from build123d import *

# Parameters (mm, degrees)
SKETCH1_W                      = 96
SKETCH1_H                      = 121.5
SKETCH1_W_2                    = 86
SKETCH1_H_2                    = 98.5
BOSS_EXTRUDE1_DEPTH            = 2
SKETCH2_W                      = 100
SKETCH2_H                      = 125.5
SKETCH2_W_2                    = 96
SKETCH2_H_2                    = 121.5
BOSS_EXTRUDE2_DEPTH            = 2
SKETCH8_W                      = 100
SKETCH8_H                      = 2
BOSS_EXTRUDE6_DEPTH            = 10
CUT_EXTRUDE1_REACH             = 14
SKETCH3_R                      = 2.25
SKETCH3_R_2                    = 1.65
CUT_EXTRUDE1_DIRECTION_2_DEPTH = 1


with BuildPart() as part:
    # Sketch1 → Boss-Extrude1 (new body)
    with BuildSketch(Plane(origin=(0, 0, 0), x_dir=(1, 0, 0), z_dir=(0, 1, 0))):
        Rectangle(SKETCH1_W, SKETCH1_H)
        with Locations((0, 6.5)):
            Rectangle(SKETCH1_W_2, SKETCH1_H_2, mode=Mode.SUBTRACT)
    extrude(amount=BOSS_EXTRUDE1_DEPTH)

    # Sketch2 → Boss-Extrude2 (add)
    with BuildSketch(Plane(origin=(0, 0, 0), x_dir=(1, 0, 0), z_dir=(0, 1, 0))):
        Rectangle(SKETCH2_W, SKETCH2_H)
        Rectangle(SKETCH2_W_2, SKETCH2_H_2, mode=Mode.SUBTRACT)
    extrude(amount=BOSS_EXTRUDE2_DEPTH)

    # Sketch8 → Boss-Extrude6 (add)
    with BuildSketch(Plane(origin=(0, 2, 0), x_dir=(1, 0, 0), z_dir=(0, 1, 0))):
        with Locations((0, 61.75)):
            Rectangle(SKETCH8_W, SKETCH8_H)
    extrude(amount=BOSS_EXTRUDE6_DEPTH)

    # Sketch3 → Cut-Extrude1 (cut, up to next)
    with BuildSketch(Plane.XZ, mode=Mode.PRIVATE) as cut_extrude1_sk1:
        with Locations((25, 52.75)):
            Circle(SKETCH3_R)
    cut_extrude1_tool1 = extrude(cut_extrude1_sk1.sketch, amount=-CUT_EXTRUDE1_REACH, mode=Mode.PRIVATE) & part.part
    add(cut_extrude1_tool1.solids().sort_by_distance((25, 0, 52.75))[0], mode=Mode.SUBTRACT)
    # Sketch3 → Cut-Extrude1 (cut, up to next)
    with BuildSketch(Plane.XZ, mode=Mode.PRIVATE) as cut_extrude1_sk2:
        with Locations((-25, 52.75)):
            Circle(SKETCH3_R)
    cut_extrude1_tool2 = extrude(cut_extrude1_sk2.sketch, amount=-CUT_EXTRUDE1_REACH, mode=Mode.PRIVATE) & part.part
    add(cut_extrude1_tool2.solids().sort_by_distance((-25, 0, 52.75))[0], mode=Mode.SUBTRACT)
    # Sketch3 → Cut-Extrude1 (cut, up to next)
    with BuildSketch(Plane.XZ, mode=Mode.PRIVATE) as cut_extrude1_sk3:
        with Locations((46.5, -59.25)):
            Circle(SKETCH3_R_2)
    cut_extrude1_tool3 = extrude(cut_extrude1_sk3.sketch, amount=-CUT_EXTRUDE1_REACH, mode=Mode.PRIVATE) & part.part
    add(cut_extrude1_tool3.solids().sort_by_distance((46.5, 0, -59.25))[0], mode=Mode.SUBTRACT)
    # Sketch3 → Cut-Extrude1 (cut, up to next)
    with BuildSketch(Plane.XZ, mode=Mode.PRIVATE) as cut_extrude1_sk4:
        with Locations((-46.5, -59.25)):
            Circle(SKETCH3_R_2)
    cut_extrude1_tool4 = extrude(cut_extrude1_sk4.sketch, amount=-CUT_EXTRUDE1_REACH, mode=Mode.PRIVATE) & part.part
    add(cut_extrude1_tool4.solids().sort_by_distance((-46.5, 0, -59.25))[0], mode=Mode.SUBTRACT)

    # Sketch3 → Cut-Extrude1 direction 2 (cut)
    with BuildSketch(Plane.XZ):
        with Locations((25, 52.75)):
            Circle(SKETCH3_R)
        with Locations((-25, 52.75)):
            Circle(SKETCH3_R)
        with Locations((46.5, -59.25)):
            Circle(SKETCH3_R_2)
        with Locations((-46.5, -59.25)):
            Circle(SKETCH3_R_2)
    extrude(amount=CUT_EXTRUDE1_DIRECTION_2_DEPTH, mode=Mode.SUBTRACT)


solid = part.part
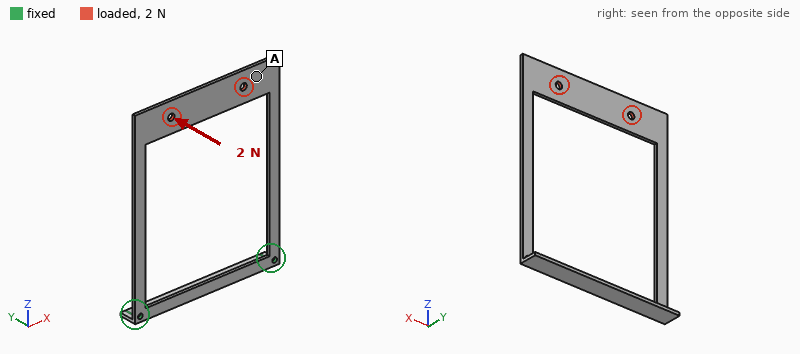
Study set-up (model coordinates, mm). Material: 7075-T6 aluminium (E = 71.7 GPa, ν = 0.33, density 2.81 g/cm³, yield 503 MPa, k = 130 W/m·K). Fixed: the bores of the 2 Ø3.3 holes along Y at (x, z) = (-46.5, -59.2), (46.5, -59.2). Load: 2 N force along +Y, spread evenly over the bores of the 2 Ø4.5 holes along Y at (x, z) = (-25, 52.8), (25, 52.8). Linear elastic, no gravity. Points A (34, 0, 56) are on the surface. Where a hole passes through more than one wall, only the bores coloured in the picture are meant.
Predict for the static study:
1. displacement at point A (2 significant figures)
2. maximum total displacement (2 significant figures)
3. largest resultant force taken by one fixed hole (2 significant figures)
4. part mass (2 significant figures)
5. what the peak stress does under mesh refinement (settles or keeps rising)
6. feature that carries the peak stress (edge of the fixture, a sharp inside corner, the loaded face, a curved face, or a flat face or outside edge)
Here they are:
1.4 mm
1.5 mm
1.0 N
28 g
keeps rising
edge of the fixture
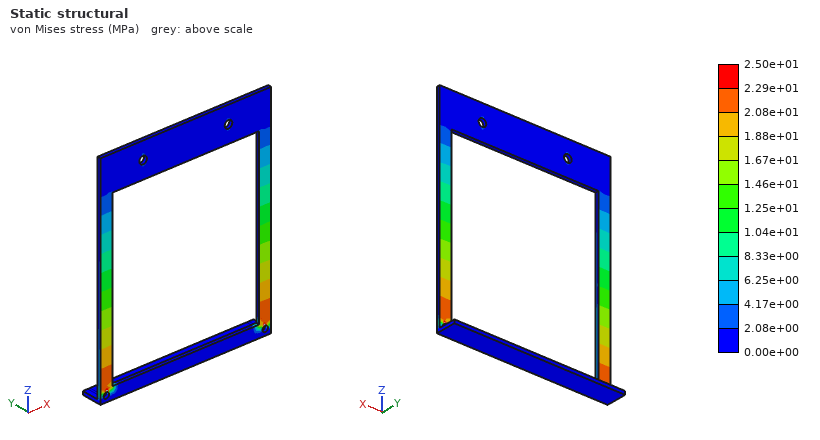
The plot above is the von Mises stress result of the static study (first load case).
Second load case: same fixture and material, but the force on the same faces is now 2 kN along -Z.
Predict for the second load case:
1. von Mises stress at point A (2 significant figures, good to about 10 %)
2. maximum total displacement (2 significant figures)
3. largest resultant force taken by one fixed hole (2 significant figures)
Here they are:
66 MPa
0.34 mm
1.0 kN
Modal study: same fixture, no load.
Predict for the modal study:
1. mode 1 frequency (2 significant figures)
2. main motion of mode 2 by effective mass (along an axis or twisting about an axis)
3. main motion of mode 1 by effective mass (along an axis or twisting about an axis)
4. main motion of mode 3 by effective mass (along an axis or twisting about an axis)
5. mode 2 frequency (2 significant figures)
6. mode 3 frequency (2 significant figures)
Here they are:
55 Hz
twisting about Z
along Y
along X
180 Hz
380 Hz
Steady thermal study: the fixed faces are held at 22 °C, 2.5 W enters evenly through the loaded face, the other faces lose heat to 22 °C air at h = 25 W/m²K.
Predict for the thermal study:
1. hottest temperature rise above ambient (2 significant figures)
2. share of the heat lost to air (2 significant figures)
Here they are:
17 K
87 %
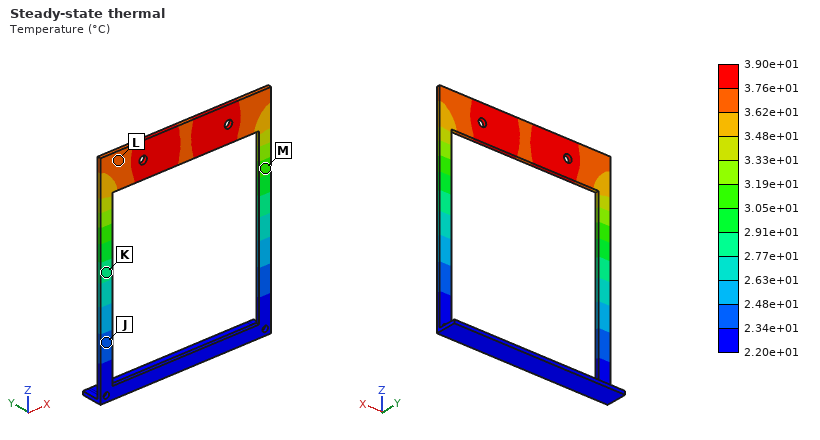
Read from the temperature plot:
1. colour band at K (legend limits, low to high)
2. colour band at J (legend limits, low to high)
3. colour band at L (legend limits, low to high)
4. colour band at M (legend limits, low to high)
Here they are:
2.77e+01 to 2.91e+01 °C
2.34e+01 to 2.48e+01 °C
3.62e+01 to 3.76e+01 °C
3.05e+01 to 3.19e+01 °C
